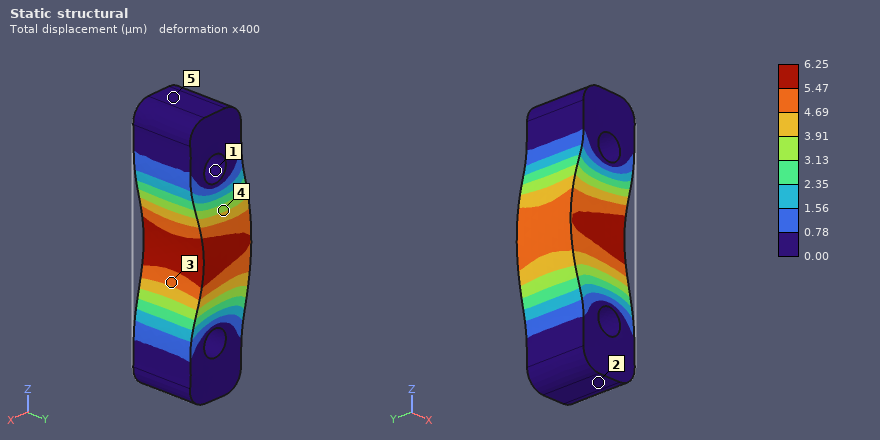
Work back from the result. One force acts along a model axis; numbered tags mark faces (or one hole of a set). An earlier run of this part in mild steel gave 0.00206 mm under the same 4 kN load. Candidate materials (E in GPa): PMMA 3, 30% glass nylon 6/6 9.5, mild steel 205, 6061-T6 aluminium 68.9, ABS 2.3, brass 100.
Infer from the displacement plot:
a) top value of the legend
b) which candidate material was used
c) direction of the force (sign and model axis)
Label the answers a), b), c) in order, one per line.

a) 6.25 µm
b) 6061-T6 aluminium
c) -X
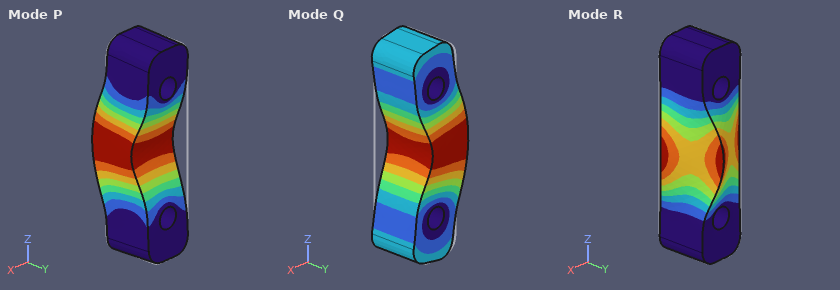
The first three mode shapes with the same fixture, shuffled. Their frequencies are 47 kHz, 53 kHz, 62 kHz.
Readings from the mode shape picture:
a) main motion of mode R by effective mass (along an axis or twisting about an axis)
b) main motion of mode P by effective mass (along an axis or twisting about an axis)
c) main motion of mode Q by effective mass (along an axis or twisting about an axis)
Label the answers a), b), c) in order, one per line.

a) twisting about Z
b) along Y
c) along X
